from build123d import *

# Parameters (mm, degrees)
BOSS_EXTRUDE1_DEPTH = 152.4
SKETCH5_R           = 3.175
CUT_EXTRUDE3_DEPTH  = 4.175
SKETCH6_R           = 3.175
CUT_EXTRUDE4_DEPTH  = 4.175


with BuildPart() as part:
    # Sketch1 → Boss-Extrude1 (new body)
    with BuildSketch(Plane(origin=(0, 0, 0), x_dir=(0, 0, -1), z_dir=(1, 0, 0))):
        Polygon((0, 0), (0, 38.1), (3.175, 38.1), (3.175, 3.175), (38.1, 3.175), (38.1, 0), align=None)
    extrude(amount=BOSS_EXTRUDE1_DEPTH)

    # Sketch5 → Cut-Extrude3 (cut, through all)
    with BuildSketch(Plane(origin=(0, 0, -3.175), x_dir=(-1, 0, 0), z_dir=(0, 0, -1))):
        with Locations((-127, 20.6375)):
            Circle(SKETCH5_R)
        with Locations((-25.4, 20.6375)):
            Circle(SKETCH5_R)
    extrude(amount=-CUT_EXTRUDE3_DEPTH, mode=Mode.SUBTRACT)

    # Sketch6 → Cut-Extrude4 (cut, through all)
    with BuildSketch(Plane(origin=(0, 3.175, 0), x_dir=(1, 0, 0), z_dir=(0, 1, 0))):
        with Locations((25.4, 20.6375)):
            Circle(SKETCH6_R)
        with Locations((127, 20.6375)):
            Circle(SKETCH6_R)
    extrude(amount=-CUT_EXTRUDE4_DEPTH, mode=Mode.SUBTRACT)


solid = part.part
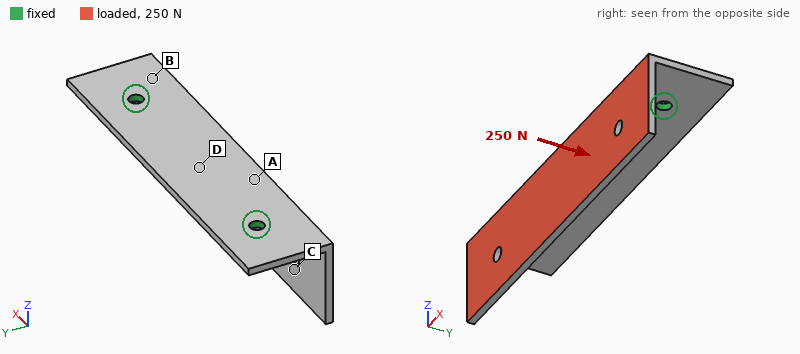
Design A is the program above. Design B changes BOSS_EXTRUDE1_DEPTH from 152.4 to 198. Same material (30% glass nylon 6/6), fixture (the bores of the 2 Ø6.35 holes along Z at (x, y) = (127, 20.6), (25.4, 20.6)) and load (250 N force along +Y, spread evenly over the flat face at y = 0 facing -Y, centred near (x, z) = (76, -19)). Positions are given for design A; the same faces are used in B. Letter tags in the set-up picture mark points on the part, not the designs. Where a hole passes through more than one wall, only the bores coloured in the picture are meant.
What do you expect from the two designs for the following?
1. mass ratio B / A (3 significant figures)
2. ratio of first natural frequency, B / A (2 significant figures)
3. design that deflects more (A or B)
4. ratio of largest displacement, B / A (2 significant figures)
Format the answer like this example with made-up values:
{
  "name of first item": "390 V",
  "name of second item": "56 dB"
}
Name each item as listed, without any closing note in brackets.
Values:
{
  "mass ratio B / A": "1.30",
  "ratio of first natural frequency, B / A": "0.86",
  "design that deflects more": "B",
  "ratio of largest displacement, B / A": "1.2"
}
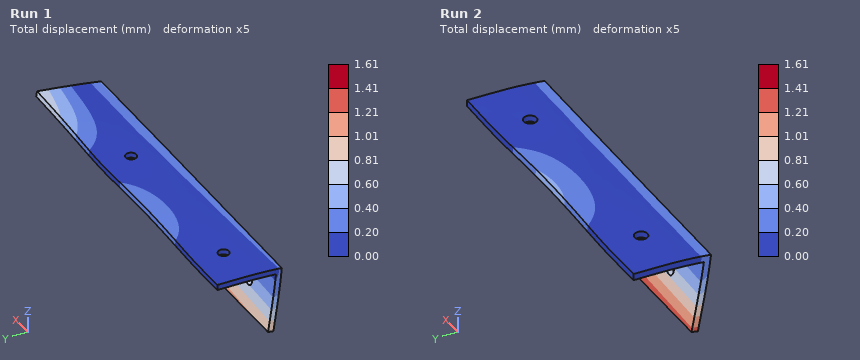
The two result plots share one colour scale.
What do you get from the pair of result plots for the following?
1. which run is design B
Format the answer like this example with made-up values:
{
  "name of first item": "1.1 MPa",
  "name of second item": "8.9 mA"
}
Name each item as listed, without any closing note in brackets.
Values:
{
  "which run is design B": "Run 1"
}
